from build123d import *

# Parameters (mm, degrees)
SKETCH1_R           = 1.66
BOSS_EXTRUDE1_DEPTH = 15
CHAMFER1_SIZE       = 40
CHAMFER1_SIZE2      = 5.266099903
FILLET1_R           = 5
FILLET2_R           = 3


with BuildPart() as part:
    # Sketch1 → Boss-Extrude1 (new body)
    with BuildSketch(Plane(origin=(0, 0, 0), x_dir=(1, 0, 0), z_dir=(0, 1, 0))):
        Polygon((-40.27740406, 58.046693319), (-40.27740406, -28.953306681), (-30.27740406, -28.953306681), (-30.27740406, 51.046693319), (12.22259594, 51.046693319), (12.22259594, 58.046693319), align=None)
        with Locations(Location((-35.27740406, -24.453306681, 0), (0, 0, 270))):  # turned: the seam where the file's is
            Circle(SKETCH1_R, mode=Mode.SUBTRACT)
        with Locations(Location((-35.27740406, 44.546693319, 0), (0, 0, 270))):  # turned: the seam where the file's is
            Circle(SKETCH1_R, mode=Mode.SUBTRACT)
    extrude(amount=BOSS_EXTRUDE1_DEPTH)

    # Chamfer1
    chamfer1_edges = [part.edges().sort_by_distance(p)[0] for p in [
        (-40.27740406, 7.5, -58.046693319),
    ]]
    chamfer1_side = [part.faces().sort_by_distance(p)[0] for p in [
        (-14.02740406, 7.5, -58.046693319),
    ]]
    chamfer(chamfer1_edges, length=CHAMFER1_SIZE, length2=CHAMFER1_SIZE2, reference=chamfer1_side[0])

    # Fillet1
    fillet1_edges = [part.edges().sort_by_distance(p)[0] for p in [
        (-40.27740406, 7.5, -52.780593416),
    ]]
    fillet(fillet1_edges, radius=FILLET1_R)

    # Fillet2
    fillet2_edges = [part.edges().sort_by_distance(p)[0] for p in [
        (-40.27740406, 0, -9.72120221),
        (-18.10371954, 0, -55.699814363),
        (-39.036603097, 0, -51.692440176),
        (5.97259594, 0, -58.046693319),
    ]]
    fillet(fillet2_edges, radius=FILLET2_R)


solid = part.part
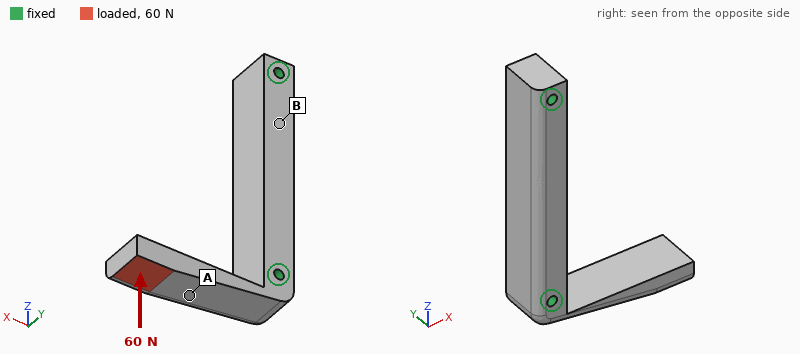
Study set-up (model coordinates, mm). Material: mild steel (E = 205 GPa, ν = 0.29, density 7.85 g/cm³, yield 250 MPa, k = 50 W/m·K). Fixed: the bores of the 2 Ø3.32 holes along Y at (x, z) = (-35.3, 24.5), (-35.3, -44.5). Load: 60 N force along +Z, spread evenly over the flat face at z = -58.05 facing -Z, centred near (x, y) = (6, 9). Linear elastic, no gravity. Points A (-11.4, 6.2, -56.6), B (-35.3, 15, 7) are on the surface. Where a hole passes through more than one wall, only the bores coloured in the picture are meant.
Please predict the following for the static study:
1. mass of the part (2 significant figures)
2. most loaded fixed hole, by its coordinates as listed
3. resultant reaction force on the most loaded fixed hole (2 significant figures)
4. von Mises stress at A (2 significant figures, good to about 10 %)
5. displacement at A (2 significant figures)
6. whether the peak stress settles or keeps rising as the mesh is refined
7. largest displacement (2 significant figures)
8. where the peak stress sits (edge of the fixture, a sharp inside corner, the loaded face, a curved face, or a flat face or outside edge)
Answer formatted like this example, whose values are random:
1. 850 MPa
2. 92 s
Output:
1. 120 g
2. (-35.3, -44.5)
3. 59 N
4. 15 MPa
5. 0.042 mm
6. keeps rising
7. 0.11 mm
8. a sharp inside corner
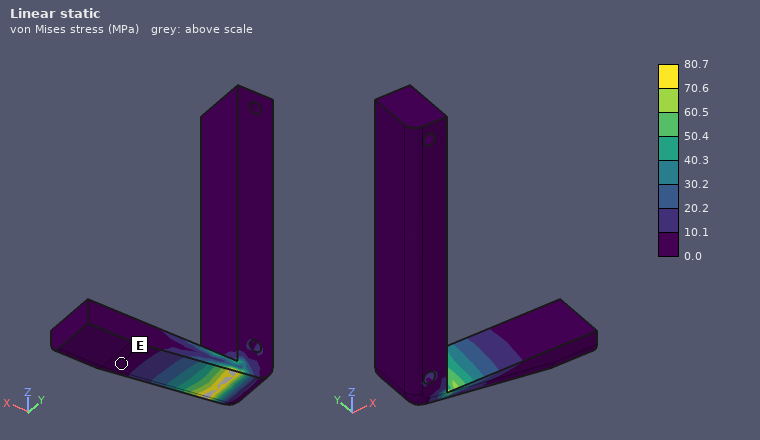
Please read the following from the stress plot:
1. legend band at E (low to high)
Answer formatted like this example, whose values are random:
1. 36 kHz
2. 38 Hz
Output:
1. 0.0 to 10.1 MPa
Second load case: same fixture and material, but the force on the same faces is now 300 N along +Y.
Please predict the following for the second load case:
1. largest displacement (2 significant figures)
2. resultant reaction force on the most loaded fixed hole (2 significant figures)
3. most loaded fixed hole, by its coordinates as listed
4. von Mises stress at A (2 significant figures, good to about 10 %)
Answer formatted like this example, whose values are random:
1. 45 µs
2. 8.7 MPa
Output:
1. 61 µm
2. 300 N
3. (-35.3, -44.5)
4. 24 MPa
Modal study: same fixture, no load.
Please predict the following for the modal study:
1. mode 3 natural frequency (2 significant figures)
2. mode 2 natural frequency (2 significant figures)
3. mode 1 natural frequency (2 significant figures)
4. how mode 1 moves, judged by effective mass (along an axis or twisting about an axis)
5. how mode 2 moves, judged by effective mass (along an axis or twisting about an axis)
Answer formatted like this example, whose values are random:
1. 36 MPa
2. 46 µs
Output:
1. 7600 Hz
2. 3200 Hz
3. 1100 Hz
4. along Z
5. along Y
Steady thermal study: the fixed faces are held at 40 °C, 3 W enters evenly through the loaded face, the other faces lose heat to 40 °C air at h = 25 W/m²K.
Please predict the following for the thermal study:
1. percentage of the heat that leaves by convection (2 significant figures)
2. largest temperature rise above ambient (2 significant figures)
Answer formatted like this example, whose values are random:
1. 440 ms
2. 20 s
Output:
1. 27 %
2. 29 K
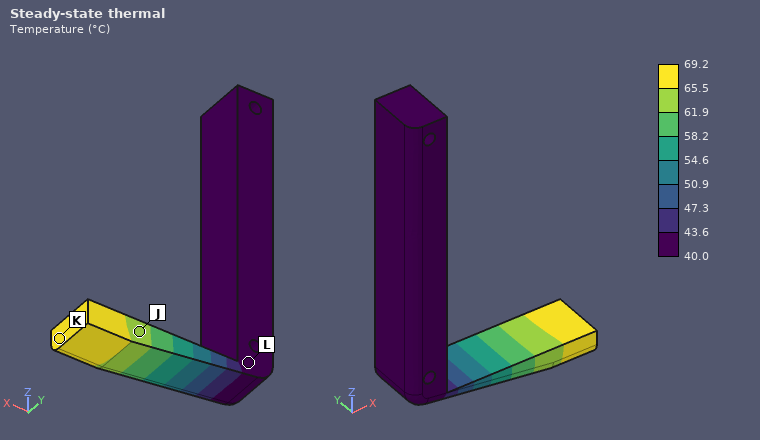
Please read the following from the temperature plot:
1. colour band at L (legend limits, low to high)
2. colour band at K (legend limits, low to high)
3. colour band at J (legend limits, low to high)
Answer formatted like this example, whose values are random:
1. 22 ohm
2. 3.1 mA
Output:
1. 40.0 to 43.6 °C
2. 65.5 to 69.2 °C
3. 61.9 to 65.5 °C
